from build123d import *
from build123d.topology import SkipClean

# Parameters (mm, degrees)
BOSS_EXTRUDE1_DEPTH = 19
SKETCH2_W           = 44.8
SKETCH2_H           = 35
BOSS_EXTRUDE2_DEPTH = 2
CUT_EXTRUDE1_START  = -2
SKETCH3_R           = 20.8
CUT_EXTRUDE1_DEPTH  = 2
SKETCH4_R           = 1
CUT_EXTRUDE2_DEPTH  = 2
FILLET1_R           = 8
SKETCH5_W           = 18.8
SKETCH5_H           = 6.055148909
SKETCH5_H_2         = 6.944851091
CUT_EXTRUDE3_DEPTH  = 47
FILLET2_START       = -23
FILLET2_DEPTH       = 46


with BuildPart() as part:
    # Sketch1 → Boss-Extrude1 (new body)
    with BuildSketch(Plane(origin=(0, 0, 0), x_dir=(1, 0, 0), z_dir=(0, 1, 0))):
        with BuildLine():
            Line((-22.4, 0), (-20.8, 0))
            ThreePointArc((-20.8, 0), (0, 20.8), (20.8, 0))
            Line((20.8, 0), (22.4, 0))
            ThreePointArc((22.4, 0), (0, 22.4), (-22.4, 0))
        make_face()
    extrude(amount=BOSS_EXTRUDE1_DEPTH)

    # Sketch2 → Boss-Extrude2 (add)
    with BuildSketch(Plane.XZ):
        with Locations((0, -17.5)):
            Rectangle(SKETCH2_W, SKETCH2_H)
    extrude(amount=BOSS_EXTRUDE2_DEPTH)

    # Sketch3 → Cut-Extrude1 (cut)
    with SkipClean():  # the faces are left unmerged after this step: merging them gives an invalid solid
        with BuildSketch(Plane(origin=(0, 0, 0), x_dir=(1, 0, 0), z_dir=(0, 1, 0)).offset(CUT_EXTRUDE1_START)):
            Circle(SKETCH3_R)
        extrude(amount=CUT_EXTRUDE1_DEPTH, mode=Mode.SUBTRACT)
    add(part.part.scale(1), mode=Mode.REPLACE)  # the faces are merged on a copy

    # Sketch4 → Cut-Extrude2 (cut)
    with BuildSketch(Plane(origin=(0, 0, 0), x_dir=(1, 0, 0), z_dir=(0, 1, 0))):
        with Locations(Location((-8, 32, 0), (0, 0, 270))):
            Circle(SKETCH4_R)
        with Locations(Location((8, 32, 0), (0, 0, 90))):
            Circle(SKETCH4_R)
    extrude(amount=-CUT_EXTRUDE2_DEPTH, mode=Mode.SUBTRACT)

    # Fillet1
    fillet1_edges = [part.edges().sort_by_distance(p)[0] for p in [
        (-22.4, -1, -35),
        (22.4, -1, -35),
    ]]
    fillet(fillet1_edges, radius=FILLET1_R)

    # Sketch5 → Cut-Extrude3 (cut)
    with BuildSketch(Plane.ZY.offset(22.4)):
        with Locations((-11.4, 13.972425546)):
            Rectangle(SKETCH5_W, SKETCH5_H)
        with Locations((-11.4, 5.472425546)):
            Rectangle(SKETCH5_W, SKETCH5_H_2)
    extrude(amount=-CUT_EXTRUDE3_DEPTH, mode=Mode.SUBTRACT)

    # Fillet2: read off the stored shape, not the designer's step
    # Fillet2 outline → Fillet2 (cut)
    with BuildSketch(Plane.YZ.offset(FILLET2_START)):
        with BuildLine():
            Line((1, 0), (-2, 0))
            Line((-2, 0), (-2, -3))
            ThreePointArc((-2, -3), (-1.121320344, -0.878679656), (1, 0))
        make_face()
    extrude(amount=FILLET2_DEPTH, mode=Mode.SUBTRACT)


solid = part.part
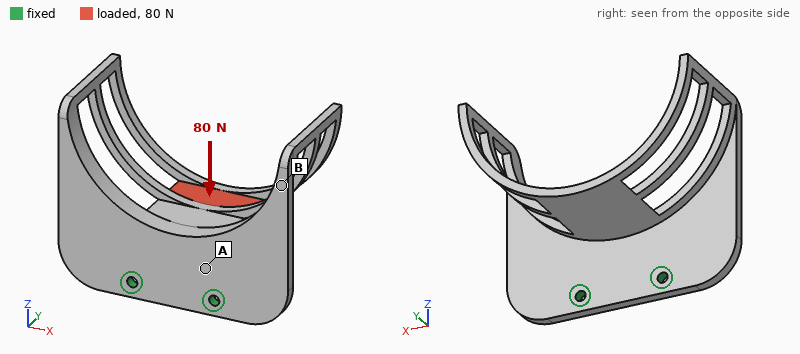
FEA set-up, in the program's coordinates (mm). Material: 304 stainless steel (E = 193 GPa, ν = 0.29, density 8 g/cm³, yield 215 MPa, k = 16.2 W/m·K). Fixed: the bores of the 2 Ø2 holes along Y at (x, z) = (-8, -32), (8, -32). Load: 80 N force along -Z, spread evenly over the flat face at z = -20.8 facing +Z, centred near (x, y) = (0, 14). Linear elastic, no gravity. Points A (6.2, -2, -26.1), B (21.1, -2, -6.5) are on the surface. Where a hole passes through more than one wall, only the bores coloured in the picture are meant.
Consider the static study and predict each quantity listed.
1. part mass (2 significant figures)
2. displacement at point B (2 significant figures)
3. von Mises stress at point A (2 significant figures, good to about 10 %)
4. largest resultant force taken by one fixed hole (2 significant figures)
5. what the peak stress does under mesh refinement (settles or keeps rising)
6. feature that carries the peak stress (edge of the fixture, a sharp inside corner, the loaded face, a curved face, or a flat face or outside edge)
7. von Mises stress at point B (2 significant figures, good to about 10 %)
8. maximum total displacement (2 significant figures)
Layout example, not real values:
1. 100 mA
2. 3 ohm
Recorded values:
1. 21 g
2. 0.076 mm
3. 45 MPa
4. 41 N
5. keeps rising
6. edge of the fixture
7. 21 MPa
8. 0.15 mm
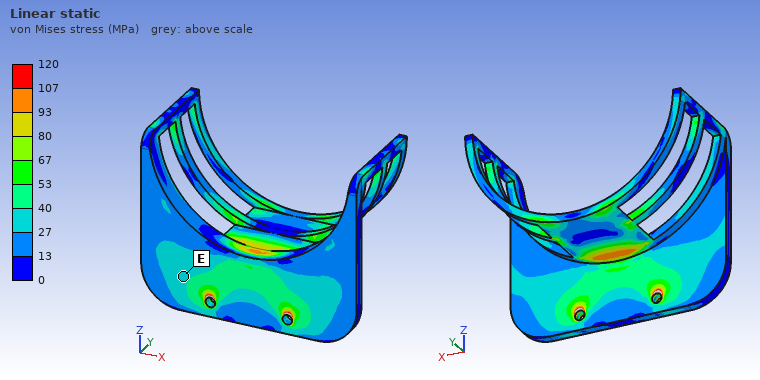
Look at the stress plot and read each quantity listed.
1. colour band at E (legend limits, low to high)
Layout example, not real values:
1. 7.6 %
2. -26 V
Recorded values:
1. 27 to 40 MPa
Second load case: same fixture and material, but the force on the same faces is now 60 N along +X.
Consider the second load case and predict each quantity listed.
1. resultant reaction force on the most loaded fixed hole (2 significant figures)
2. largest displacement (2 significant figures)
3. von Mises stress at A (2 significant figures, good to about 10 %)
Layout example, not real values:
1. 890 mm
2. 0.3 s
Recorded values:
1. 69 N
2. 31 µm
3. 18 MPa
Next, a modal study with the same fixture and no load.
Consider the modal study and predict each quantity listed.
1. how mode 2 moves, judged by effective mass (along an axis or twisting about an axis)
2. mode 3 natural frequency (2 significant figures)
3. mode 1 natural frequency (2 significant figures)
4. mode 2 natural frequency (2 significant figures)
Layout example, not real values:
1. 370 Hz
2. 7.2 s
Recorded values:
1. twisting about Z
2. 2400 Hz
3. 1400 Hz
4. 1800 Hz
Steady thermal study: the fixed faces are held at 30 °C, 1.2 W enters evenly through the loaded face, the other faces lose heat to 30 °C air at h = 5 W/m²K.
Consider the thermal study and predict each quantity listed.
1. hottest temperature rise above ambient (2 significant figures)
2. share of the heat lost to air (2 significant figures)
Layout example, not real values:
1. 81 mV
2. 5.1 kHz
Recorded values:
1. 57 K
2. 27 %
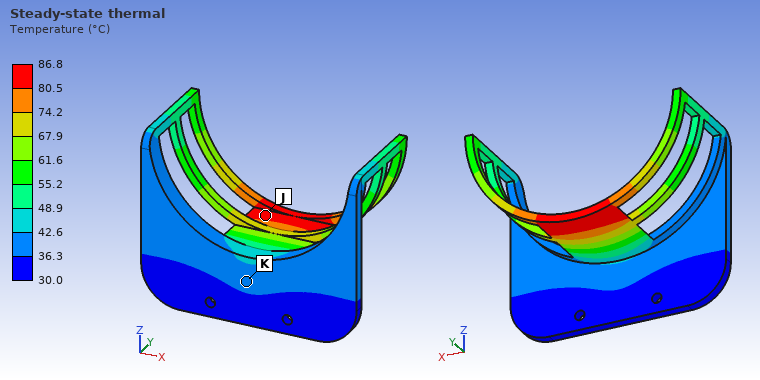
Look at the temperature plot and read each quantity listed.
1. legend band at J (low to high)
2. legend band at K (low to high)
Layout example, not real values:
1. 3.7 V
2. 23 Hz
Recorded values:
1. 80.5 to 86.8 °C
2. 36.3 to 42.6 °C
